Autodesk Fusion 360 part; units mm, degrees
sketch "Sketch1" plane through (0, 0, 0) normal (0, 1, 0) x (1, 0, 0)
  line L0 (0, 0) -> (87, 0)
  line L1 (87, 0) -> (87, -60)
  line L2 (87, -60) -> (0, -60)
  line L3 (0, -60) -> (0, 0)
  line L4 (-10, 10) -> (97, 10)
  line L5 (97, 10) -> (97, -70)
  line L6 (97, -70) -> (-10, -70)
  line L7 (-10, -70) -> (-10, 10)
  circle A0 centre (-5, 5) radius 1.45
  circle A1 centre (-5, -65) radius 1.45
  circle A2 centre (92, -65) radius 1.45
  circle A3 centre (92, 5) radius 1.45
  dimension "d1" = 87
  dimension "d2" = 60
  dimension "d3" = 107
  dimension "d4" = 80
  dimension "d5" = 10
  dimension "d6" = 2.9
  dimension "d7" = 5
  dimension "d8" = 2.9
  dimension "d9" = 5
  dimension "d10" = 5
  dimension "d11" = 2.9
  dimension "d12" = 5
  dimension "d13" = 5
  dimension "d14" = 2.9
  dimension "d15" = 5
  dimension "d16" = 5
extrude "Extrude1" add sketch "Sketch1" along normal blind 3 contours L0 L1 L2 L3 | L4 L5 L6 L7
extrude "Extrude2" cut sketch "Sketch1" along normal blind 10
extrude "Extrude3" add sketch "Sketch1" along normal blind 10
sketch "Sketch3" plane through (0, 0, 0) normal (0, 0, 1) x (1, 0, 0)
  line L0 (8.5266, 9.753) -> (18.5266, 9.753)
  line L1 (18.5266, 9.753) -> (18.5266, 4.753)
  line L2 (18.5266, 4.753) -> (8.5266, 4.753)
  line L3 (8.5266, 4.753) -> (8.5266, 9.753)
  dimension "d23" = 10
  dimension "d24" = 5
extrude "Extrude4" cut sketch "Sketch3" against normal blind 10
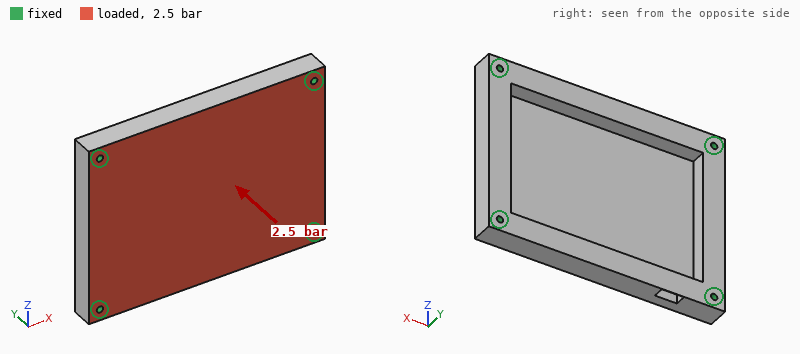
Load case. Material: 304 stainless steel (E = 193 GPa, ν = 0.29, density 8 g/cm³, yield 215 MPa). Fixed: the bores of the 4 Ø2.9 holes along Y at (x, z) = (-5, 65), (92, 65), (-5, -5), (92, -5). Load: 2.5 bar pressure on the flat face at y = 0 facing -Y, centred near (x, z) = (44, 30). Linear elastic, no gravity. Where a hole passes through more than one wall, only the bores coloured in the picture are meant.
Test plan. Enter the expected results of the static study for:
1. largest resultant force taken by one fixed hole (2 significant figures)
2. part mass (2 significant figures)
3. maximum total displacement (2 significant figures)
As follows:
670 N
390 g
38 µm
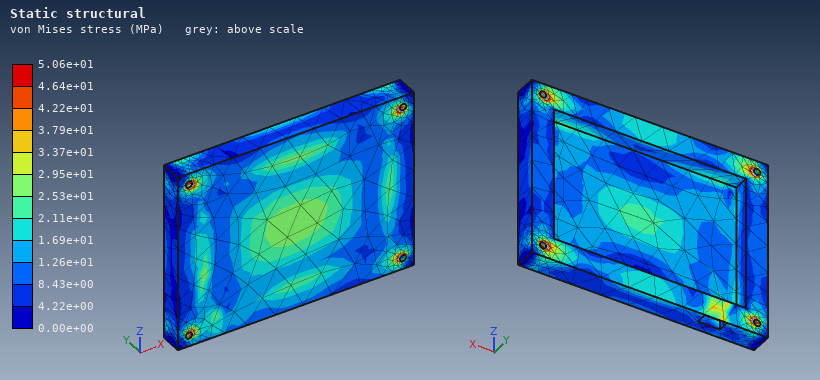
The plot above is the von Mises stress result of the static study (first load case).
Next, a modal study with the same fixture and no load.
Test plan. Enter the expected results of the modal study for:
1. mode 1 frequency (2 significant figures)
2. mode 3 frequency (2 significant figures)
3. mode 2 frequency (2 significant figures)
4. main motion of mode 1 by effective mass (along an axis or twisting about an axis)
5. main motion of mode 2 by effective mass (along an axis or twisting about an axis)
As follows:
3200 Hz
5700 Hz
4600 Hz
along Y
twisting about X
